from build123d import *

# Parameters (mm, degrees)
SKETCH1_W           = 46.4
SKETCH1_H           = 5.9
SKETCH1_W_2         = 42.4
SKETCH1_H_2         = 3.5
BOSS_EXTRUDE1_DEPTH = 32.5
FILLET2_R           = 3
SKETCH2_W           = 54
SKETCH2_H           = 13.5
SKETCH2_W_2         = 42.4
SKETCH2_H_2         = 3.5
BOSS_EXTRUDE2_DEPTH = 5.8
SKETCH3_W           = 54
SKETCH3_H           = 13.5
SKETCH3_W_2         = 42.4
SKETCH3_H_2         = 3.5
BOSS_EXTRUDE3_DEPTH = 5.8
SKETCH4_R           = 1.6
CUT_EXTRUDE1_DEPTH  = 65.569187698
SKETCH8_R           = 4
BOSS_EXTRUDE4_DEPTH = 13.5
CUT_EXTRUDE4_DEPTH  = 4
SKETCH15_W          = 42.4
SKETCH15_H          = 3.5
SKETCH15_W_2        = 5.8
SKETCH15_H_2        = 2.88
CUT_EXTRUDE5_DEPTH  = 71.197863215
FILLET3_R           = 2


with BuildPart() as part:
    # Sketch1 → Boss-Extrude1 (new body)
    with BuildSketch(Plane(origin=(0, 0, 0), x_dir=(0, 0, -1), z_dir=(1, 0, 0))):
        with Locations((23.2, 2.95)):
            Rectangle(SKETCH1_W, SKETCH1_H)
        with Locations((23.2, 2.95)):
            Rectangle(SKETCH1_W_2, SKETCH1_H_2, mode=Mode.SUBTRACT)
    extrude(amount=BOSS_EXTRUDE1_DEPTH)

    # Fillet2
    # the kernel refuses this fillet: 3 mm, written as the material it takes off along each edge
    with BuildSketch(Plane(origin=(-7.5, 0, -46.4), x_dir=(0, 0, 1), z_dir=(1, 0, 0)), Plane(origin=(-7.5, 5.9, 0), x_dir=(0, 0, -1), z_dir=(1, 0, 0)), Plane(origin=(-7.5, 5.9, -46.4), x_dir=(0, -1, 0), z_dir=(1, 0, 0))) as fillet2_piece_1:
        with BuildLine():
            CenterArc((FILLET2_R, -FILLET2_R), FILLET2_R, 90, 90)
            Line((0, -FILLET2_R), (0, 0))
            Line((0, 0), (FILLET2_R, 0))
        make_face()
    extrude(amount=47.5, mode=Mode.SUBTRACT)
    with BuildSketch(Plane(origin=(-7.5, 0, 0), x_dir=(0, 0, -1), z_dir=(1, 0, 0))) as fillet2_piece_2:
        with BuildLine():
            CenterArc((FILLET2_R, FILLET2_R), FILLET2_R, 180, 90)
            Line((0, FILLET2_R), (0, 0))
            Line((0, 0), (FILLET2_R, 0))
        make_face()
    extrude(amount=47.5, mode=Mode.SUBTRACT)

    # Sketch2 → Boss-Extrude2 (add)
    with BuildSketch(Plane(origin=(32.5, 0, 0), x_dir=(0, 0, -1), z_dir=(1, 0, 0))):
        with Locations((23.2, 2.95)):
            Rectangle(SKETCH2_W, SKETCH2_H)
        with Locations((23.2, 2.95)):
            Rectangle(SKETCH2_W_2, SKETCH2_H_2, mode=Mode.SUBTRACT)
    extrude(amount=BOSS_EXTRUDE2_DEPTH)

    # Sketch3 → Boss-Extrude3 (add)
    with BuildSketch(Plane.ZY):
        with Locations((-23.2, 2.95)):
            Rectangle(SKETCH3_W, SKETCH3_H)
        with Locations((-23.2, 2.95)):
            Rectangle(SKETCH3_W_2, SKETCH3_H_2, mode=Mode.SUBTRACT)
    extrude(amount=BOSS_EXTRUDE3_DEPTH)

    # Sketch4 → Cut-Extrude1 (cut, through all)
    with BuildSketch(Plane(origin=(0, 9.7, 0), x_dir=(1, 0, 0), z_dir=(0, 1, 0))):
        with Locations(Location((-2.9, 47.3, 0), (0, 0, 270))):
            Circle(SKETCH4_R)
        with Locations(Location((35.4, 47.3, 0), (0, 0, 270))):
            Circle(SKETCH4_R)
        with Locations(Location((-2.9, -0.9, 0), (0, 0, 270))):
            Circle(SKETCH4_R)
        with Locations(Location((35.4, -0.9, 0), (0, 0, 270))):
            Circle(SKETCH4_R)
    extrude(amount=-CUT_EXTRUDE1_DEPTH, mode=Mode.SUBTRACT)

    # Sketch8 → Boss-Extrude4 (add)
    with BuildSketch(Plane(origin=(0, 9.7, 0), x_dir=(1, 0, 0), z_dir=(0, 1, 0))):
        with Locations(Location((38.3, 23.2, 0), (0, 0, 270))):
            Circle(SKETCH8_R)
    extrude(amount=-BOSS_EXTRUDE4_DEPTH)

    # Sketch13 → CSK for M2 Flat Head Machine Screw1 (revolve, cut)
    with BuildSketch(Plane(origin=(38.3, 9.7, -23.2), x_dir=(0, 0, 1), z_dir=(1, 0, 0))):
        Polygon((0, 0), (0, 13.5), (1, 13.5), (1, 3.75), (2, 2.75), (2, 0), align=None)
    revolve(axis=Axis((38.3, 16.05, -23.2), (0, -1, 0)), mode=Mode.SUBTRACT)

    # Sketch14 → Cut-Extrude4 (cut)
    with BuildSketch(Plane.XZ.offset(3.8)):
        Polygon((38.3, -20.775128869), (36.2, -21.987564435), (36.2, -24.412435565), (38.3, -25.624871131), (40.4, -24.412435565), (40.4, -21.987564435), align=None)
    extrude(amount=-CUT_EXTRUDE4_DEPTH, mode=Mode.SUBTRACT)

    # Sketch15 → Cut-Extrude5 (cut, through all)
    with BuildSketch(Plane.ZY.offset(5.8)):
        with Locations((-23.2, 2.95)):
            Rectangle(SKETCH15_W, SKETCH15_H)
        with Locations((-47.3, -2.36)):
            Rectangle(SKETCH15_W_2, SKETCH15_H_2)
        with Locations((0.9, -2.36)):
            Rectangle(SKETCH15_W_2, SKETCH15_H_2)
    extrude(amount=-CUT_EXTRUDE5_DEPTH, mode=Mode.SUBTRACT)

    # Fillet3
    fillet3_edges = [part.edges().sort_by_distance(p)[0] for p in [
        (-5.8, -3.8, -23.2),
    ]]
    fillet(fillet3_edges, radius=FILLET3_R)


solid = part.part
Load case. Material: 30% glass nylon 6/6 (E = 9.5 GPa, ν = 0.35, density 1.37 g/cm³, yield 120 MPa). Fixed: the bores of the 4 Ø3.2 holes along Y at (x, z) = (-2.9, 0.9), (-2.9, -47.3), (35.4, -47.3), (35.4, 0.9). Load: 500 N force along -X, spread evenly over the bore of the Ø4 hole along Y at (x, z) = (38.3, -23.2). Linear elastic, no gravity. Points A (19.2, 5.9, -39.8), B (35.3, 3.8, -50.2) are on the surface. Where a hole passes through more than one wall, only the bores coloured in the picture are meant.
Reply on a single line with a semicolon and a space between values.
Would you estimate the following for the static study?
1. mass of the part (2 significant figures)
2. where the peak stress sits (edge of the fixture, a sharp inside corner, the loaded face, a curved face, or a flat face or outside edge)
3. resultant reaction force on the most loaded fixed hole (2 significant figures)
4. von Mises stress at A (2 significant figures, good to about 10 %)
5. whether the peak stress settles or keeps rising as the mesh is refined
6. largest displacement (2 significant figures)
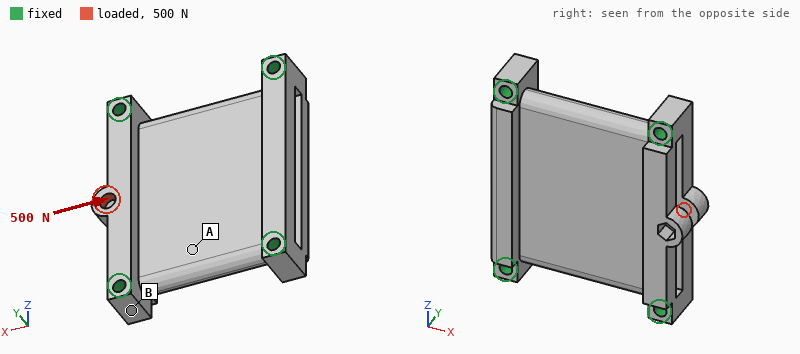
14 g; edge of the fixture; 160 N; 6.6 MPa; keeps rising; 0.26 mm
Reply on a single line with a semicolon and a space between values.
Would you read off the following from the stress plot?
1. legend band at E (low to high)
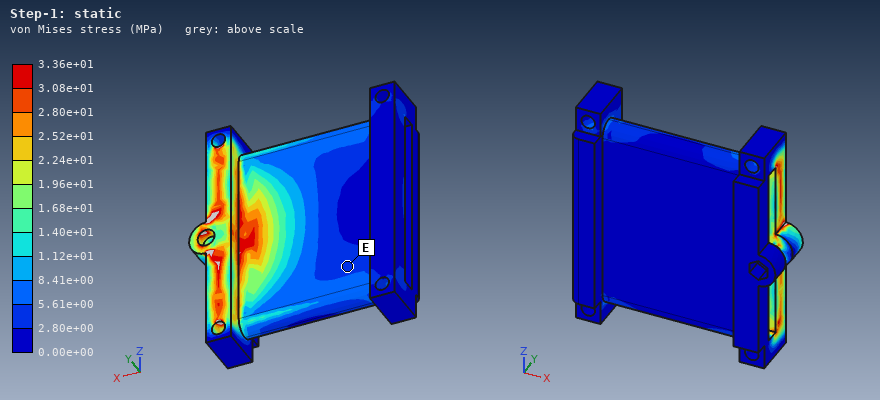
2.80e+00 to 5.61e+00 MPa
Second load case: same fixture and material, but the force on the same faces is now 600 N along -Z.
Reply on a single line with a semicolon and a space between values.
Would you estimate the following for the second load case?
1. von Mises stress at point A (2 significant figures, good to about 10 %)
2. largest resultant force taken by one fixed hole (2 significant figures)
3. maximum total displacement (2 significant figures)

3.0 MPa; 290 N; 61 µm
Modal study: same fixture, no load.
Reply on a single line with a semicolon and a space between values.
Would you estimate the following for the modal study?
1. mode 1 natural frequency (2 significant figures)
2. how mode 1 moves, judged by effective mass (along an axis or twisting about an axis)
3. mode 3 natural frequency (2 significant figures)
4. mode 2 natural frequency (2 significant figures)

3000 Hz; along Y; 4200 Hz; 3300 Hz
